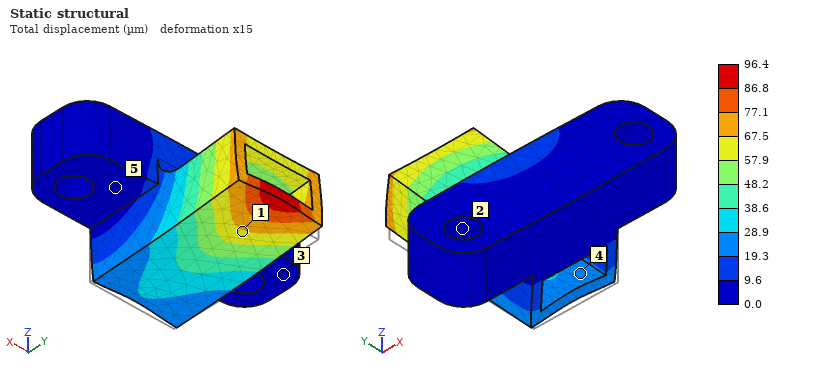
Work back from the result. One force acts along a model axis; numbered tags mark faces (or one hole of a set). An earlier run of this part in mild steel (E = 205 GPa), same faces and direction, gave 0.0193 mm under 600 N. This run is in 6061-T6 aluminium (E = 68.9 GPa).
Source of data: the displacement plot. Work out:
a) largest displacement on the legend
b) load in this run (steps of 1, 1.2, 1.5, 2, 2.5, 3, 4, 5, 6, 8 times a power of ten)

96.4 µm
1 kN
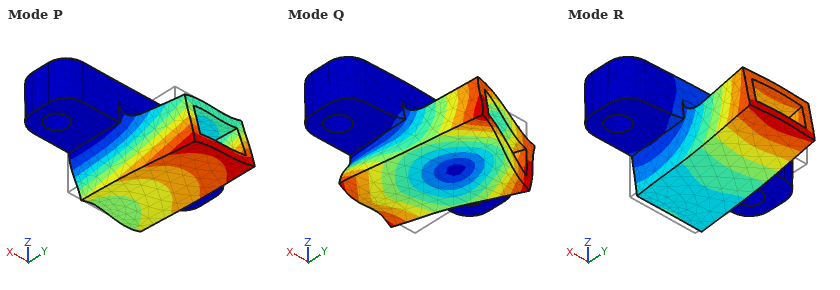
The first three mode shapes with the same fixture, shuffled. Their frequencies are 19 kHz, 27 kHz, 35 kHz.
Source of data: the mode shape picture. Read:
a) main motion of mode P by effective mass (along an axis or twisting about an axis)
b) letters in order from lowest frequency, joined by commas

along X
R, P, Q
